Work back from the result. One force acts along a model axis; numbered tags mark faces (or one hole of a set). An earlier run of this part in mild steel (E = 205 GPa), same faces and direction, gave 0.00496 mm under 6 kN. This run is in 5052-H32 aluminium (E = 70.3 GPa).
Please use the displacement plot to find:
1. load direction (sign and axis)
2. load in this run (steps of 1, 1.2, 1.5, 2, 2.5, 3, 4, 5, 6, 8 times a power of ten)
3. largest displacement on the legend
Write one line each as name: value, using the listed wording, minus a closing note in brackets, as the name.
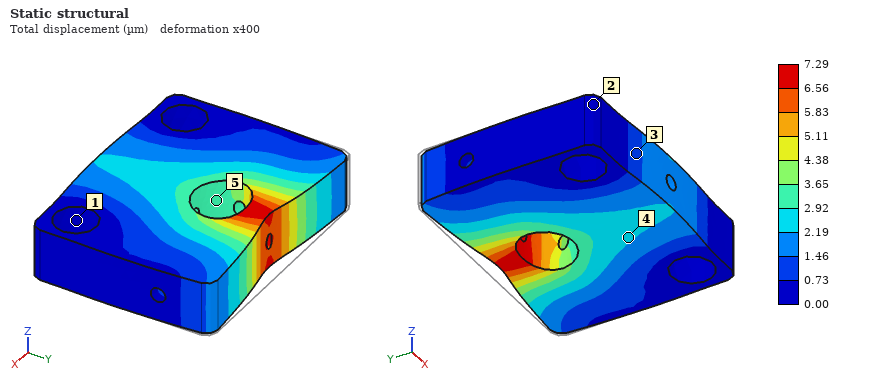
load direction: -Y
load in this run: 3 kN
largest displacement on the legend: 7.29 µm
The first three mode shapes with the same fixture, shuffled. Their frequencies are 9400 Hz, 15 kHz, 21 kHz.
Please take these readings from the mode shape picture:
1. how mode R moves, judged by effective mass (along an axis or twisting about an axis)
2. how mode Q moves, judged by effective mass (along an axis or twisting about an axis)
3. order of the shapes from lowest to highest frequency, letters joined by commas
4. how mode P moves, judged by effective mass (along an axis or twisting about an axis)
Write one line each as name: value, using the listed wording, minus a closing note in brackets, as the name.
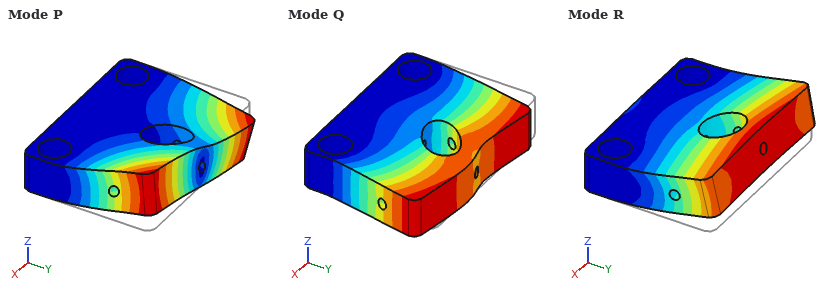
how mode R moves, judged by effective mass: along Z
how mode Q moves, judged by effective mass: along X
order of the shapes from lowest to highest frequency, letters joined by commas: R, P, Q
how mode P moves, judged by effective mass: twisting about Y
